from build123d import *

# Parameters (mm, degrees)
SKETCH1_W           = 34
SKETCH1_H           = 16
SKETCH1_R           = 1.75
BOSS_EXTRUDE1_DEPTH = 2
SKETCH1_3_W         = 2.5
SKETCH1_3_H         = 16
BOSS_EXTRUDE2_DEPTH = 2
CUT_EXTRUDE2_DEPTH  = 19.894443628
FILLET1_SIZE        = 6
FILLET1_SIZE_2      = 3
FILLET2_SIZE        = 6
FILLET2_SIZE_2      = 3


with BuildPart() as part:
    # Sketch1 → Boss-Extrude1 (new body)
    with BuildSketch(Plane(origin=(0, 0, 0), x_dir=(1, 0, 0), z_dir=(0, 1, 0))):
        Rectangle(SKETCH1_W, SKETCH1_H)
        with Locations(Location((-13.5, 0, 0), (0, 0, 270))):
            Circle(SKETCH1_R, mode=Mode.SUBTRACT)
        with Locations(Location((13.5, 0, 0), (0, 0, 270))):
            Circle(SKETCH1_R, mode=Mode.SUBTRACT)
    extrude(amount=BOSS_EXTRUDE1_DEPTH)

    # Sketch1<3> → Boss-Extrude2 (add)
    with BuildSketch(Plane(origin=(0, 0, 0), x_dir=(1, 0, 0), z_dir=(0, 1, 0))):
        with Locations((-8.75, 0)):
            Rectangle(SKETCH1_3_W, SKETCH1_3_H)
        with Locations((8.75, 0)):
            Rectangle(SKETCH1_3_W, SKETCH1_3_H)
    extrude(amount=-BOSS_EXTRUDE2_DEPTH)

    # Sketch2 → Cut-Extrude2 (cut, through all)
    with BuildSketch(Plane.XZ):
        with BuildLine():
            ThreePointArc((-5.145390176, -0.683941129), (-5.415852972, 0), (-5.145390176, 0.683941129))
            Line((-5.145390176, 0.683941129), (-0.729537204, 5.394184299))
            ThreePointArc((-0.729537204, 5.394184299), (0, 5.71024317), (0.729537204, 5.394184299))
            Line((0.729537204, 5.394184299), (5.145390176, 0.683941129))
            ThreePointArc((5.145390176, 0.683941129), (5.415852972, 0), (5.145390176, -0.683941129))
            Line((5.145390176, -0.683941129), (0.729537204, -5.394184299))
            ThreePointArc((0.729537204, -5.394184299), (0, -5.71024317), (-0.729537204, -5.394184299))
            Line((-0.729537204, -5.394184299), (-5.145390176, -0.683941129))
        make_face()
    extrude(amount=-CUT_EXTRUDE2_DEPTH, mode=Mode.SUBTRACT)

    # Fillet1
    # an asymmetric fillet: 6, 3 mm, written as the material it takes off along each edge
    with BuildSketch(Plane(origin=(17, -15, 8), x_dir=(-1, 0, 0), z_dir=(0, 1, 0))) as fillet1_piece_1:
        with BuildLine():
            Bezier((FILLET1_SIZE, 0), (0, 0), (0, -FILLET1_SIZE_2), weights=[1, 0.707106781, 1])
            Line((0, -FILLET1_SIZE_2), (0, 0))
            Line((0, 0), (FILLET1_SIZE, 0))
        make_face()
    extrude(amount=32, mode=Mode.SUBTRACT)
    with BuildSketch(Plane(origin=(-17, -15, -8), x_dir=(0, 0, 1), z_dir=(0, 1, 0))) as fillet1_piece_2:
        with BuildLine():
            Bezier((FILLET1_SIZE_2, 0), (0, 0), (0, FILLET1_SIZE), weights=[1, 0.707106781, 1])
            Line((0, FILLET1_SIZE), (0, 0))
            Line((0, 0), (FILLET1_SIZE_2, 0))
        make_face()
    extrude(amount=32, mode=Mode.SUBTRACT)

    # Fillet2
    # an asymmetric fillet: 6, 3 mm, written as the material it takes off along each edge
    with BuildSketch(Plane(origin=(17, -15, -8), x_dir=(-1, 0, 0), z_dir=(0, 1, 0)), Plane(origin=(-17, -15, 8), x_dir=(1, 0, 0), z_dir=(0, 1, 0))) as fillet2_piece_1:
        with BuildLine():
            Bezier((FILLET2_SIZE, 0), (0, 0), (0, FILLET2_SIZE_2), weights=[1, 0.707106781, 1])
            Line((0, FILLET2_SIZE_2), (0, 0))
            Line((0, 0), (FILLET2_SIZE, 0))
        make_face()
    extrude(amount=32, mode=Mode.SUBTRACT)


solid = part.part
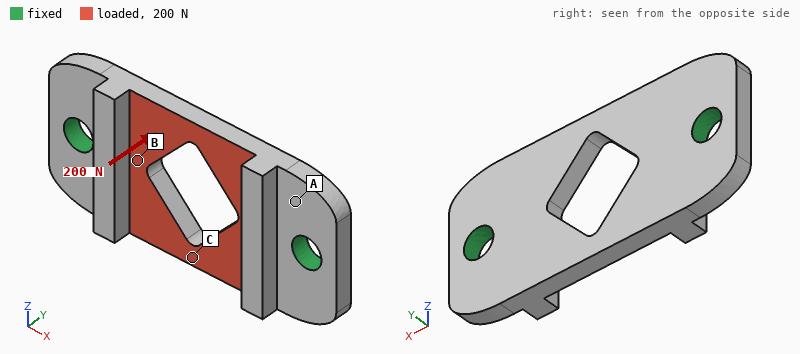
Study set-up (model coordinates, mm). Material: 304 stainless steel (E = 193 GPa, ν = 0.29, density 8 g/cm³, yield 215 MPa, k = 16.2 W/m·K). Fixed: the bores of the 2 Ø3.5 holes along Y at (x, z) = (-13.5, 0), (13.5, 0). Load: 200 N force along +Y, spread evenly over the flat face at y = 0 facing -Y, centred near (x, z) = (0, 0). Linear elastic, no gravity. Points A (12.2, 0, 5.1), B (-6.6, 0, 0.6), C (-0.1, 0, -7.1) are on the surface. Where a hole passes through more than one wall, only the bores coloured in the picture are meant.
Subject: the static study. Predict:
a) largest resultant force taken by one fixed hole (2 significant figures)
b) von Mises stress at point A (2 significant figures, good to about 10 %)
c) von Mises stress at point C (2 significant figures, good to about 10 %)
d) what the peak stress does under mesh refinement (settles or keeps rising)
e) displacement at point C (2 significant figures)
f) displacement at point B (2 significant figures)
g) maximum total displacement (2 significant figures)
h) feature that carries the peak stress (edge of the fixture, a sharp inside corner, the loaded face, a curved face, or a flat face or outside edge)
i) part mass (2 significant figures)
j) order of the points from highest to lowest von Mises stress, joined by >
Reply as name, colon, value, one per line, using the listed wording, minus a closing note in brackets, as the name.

largest resultant force taken by one fixed hole: 100 N
von Mises stress at point A: 26 MPa
von Mises stress at point C: 54 MPa
what the peak stress does under mesh refinement: keeps rising
displacement at point C: 10 µm
displacement at point B: 4.7 µm
maximum total displacement: 10 µm
feature that carries the peak stress: edge of the fixture
part mass: 8.3 g
order of the points from highest to lowest von Mises stress, joined by >: C > A > B
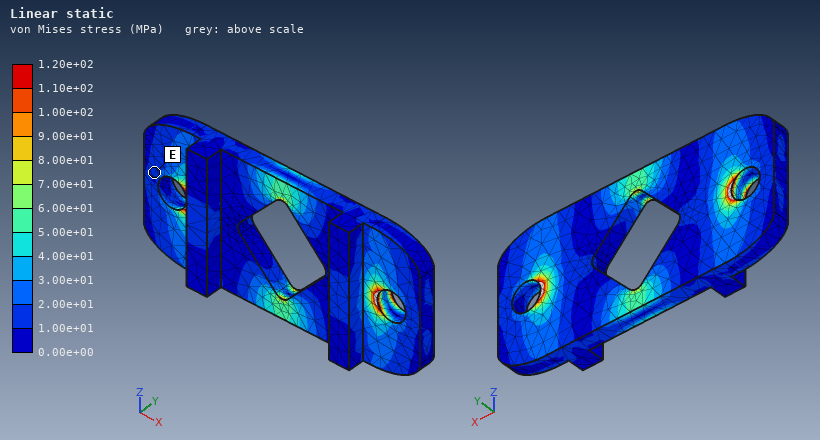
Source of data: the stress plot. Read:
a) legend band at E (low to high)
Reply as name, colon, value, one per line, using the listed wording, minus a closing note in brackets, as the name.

legend band at E: 1.00e+01 to 2.00e+01 MPa
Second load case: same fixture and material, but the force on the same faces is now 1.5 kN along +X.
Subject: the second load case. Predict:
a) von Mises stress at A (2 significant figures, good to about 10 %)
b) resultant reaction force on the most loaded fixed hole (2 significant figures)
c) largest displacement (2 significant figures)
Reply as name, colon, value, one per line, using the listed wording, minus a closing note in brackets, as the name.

von Mises stress at A: 16 MPa
resultant reaction force on the most loaded fixed hole: 750 N
largest displacement: 2.2 µm
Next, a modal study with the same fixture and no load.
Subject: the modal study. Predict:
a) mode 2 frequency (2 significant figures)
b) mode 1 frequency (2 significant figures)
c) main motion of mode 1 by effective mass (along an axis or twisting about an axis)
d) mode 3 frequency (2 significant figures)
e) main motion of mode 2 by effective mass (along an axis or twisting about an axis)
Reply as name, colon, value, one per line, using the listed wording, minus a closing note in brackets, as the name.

mode 2 frequency: 15 kHz
mode 1 frequency: 14 kHz
main motion of mode 1 by effective mass: along Y
mode 3 frequency: 26 kHz
main motion of mode 2 by effective mass: twisting about X
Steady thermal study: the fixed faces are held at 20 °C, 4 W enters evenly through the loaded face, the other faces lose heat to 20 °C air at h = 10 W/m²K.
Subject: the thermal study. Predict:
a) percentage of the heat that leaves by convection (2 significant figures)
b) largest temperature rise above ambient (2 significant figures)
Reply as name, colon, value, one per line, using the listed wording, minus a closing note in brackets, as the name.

percentage of the heat that leaves by convection: 4.9 %
largest temperature rise above ambient: 40 K
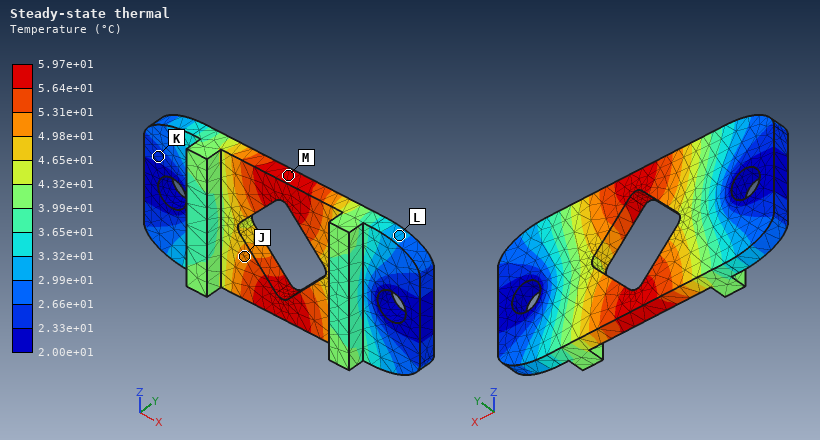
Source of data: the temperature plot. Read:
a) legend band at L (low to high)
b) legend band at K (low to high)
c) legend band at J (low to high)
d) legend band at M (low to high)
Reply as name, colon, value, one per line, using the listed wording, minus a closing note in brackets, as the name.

legend band at L: 2.99e+01 to 3.32e+01 °C
legend band at K: 2.33e+01 to 2.66e+01 °C
legend band at J: 4.98e+01 to 5.31e+01 °C
legend band at M: 5.64e+01 to 5.97e+01 °C
